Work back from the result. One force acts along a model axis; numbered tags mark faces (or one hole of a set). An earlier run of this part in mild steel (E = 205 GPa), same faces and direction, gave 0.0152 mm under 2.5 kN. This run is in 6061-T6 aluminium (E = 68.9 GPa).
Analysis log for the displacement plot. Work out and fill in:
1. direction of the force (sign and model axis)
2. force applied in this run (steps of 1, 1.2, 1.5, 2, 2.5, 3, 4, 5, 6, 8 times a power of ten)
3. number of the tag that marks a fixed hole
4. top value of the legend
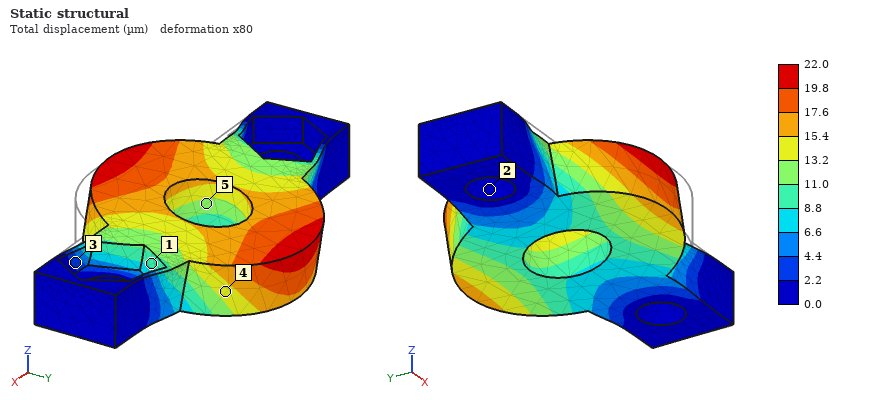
+Y
1.2 kN
2
22.0 µm
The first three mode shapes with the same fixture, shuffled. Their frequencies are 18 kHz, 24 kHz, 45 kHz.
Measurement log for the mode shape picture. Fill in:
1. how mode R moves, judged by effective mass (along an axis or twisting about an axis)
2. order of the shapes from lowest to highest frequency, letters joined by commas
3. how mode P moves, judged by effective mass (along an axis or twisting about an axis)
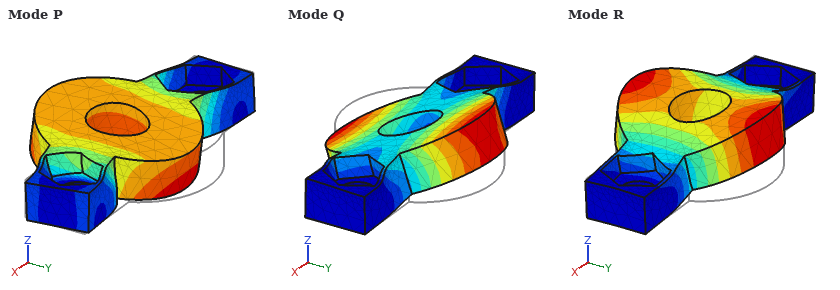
along Z
Q, R, P
along Y
